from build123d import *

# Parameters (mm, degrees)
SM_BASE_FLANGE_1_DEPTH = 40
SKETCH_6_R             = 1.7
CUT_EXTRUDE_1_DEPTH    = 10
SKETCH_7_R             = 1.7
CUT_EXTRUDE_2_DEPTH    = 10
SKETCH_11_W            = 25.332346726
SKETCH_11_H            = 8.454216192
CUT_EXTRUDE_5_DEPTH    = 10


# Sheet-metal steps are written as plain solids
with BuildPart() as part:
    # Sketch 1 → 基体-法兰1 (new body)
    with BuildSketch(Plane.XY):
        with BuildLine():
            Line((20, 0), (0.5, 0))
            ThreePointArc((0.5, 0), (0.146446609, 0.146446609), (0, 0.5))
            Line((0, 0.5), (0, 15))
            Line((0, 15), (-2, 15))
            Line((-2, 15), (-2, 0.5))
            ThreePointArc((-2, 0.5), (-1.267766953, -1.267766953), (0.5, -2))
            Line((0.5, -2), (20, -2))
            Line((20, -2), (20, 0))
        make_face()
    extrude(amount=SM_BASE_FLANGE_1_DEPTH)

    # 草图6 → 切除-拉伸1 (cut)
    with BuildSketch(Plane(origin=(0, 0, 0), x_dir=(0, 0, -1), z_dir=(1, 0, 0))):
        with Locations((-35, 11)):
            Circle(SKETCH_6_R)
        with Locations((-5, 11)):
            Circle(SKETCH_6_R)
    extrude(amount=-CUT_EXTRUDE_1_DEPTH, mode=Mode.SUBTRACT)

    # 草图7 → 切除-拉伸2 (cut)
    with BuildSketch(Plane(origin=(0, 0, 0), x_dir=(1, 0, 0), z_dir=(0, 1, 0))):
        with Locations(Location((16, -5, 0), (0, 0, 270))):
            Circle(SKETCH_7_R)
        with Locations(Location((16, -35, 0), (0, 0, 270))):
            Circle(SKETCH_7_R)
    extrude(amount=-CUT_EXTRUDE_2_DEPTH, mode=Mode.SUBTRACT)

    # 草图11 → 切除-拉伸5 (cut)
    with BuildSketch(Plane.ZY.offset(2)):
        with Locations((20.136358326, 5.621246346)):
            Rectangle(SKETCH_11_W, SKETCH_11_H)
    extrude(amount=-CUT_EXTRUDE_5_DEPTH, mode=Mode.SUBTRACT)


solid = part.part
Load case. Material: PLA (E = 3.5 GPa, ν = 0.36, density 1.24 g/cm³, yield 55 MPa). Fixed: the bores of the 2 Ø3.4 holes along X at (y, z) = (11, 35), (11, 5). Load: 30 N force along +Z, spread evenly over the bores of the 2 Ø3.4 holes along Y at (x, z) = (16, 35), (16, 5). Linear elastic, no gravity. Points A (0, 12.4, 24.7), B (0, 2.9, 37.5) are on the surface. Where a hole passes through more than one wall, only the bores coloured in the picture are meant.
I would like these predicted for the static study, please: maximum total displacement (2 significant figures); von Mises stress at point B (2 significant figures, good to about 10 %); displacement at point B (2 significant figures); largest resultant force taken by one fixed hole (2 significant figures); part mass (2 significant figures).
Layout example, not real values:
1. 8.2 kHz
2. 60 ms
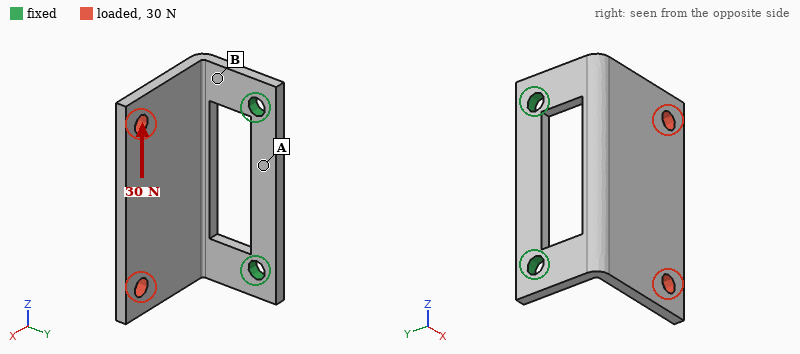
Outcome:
1. 0.44 mm
2. 6.8 MPa
3. 0.12 mm
4. 22 N
5. 3.0 g
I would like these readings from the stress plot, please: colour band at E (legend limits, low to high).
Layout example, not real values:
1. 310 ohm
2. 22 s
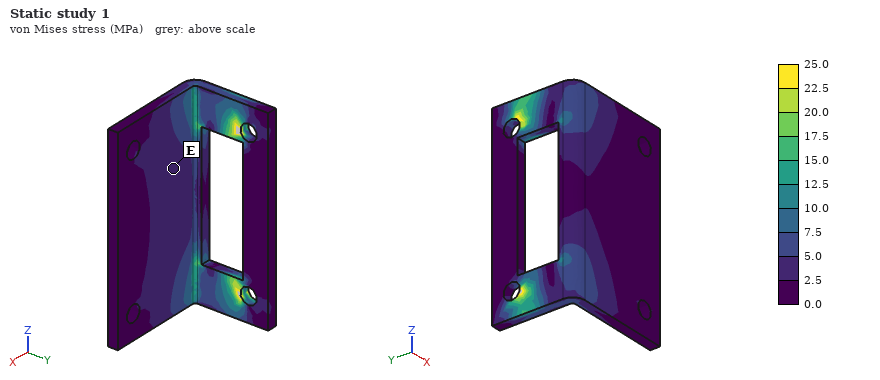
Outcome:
1. 2.5 to 5.0 MPa
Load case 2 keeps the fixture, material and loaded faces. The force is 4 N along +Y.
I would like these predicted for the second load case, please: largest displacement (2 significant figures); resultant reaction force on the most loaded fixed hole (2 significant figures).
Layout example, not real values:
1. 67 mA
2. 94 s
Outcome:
1. 0.57 mm
2. 2.0 N
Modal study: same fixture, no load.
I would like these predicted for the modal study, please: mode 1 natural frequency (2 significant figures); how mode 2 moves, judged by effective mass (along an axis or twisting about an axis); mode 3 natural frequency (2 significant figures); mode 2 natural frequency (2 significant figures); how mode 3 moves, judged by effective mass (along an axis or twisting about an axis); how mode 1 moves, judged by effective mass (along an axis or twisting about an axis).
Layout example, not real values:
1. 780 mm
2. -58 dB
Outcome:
1. 440 Hz
2. along Z
3. 1600 Hz
4. 1100 Hz
5. along X
6. along Y
